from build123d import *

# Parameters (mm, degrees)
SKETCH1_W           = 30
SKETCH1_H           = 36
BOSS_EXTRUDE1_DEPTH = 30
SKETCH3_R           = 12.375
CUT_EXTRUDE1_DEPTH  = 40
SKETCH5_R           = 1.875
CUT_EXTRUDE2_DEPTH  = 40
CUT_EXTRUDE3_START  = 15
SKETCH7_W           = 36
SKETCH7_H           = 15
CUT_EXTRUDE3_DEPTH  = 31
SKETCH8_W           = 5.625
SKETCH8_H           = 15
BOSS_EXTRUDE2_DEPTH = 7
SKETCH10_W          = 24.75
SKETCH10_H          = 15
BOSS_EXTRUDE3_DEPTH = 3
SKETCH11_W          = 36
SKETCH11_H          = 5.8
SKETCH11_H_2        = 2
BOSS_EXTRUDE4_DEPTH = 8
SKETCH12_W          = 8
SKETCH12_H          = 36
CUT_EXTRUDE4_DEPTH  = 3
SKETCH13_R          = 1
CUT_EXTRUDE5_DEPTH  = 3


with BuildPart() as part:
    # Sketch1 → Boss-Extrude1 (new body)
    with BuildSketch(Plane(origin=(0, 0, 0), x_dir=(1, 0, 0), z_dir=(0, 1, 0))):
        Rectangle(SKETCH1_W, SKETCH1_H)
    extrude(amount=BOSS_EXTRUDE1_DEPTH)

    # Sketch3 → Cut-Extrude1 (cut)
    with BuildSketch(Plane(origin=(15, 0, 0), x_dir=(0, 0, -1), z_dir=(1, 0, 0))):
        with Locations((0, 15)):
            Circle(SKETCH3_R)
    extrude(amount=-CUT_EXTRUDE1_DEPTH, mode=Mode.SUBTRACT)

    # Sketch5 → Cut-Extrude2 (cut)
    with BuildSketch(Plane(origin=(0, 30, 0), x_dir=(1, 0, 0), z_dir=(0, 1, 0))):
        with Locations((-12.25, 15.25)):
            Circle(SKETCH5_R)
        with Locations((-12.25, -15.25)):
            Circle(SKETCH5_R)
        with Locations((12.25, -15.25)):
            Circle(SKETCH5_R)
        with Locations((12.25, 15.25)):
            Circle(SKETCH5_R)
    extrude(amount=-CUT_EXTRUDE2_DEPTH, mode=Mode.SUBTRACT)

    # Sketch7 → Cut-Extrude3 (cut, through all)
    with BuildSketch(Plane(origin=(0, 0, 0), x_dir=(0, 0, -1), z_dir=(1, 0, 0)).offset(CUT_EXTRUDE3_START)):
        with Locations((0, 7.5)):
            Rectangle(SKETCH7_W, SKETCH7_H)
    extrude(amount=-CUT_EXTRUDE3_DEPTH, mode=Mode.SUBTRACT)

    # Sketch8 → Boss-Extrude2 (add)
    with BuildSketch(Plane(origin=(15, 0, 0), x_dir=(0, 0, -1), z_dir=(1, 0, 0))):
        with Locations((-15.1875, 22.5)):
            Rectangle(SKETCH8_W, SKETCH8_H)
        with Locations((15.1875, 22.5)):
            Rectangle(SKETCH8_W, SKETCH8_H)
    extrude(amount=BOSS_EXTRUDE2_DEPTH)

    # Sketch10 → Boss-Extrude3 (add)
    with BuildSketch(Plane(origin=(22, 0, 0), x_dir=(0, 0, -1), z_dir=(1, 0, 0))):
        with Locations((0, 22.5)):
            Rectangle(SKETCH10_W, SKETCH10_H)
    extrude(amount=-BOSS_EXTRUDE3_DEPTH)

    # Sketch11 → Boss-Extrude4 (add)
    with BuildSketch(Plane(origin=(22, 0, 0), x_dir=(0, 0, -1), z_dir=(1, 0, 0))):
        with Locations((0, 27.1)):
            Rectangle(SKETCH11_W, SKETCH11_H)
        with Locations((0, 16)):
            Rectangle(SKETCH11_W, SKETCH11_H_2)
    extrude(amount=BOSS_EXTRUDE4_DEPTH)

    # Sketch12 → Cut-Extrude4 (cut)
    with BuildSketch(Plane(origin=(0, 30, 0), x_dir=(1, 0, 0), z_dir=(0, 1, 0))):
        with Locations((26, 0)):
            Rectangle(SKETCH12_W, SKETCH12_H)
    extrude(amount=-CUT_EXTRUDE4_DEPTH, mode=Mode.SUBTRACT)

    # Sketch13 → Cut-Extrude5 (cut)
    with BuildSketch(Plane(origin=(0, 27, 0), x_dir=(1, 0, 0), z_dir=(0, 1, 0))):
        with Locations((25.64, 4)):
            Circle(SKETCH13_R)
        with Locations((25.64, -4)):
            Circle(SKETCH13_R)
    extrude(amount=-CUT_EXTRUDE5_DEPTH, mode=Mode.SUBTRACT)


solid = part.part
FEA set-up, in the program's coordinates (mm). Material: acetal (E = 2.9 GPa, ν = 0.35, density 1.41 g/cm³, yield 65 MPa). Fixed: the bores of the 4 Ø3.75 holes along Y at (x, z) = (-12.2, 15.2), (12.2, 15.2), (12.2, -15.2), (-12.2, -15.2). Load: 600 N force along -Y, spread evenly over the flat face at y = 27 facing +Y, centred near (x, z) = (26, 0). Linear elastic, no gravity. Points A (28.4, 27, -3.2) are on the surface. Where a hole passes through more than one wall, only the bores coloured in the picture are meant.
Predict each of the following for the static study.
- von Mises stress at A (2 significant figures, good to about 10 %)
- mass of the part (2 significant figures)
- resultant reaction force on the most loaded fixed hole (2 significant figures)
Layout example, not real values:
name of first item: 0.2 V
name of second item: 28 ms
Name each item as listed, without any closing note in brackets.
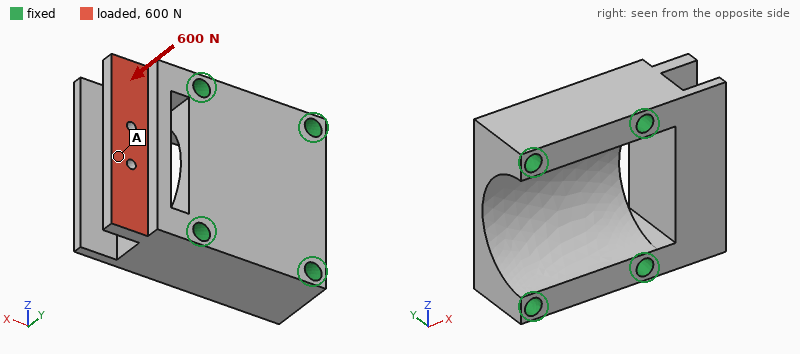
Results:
von Mises stress at A: 4.9 MPa
mass of the part: 17 g
resultant reaction force on the most loaded fixed hole: 300 N
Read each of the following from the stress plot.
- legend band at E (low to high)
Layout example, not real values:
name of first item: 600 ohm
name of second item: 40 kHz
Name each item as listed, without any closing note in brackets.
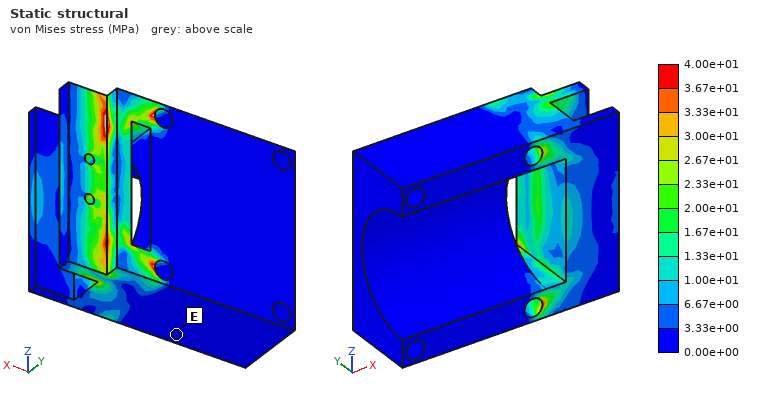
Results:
legend band at E: 0.00e+00 to 3.33e+00 MPa
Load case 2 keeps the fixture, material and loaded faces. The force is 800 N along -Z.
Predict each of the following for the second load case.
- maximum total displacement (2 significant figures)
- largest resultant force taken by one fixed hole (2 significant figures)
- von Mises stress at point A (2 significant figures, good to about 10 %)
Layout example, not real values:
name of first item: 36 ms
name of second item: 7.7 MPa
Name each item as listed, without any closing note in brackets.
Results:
maximum total displacement: 0.22 mm
largest resultant force taken by one fixed hole: 480 N
von Mises stress at point A: 11 MPa
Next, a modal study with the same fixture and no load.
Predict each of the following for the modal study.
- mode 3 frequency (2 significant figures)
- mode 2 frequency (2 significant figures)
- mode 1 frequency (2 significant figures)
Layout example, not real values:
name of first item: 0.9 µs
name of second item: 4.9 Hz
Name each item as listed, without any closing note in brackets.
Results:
mode 3 frequency: 6000 Hz
mode 2 frequency: 5800 Hz
mode 1 frequency: 4500 Hz
